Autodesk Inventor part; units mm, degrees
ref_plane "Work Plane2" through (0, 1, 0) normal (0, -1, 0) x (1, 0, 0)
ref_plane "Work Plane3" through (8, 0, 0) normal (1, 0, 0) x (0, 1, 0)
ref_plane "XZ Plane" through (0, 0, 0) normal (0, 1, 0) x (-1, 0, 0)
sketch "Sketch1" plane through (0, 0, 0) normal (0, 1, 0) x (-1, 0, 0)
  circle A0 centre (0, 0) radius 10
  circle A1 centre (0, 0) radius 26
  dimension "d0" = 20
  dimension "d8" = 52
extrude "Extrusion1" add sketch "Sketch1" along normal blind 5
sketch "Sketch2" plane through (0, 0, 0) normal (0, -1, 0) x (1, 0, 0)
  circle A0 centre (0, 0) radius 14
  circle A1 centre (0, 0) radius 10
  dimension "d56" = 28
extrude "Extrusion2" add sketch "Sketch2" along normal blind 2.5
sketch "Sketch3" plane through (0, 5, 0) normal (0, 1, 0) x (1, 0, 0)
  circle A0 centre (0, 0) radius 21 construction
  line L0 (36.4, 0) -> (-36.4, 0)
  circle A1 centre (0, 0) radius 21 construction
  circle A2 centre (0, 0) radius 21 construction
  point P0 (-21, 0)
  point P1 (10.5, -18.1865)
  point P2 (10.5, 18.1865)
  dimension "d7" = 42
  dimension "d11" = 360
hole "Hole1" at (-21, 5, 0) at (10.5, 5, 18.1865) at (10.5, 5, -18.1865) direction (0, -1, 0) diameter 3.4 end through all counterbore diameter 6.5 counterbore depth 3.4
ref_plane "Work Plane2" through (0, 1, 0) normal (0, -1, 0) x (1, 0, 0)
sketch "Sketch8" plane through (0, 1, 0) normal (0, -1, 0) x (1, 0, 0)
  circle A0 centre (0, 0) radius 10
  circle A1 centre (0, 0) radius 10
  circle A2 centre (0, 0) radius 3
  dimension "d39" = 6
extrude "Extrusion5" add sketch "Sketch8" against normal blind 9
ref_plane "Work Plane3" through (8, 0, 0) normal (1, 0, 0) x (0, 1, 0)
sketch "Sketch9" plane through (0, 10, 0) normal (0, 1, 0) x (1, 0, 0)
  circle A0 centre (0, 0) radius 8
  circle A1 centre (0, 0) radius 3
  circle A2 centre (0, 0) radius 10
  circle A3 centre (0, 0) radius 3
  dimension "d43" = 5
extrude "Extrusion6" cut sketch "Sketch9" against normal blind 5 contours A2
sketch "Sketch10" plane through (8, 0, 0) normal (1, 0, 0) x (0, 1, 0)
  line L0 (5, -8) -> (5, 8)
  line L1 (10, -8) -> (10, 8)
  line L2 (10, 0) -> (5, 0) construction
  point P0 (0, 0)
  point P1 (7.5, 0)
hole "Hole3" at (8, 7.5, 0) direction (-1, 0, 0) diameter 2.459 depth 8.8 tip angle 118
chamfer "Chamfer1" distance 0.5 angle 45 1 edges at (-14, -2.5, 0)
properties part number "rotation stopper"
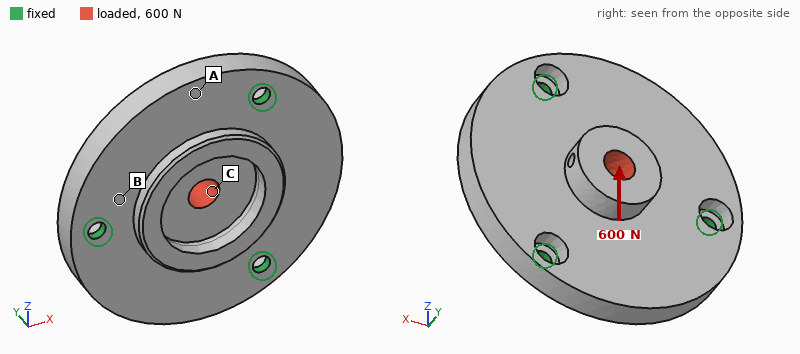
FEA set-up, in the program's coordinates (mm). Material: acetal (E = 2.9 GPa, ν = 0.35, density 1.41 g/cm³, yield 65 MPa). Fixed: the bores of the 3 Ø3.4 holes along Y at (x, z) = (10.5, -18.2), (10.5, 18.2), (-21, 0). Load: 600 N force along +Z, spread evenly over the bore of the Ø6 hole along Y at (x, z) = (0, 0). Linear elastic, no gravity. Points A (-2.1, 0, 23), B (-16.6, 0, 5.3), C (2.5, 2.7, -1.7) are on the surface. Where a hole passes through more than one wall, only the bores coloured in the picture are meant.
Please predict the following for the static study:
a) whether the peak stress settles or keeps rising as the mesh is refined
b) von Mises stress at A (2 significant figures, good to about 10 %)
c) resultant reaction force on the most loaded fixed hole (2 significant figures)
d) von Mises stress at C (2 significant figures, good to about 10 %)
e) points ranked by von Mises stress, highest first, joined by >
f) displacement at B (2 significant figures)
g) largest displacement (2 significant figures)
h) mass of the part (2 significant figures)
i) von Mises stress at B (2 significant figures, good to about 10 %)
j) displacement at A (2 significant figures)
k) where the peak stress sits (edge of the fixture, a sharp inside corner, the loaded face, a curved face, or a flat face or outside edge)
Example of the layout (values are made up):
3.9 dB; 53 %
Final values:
keeps rising; 2.0 MPa; 250 N; 6.2 MPa; C > B > A; 0.028 mm; 0.11 mm; 16 g; 3.8 MPa; 0.069 mm; edge of the fixture
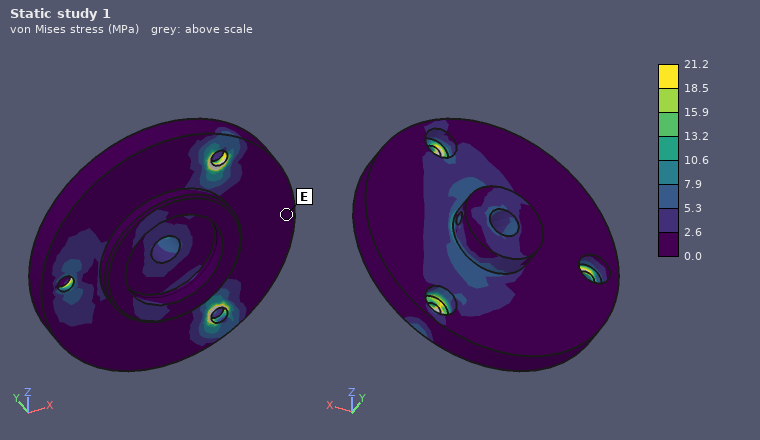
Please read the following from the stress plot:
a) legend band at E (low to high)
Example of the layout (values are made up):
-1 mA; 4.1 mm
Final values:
0.0 to 2.6 MPa
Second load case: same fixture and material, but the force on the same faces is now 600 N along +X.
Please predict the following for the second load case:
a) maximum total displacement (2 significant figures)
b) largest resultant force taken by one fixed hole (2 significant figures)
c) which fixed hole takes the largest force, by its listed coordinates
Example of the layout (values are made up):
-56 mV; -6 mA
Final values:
0.12 mm; 270 N; (-21, 0)
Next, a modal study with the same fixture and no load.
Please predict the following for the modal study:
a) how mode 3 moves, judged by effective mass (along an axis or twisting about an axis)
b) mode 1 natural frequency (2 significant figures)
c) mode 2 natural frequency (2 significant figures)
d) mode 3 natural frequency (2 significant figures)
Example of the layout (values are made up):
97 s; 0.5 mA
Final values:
along Y; 2500 Hz; 2500 Hz; 3000 Hz
